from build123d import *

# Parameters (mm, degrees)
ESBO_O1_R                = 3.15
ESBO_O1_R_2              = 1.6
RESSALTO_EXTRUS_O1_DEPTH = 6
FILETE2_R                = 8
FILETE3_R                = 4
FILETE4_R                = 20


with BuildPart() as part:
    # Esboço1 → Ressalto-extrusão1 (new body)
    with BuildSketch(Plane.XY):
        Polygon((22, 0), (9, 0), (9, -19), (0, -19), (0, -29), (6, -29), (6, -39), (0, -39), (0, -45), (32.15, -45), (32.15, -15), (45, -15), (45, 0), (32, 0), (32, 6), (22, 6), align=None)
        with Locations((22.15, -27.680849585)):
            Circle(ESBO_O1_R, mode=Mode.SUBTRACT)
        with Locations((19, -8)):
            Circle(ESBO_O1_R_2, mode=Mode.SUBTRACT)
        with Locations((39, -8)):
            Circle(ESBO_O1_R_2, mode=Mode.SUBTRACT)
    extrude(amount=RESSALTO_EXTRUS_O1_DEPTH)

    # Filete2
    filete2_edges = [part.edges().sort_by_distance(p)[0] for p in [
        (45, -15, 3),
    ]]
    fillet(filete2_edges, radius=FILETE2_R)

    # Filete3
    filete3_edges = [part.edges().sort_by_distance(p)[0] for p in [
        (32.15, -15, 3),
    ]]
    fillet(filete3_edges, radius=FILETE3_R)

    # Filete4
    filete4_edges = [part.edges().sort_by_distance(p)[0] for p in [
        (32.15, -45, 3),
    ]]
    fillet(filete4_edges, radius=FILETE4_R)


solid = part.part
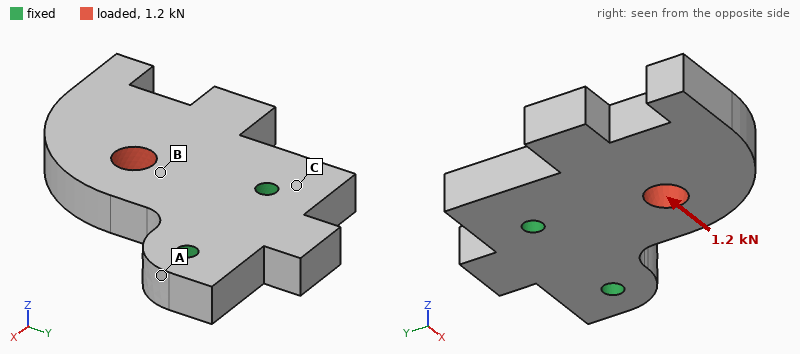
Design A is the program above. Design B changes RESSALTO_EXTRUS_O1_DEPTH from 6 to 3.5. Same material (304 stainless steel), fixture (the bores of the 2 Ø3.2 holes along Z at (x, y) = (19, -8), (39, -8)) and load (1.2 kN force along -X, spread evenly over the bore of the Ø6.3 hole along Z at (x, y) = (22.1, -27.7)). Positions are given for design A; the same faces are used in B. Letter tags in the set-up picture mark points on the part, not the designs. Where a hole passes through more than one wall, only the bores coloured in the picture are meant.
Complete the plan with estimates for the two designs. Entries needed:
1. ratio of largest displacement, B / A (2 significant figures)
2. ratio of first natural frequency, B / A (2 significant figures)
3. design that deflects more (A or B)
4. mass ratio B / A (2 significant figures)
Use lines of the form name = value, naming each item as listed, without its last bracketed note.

ratio of largest displacement, B / A = 1.7
ratio of first natural frequency, B / A = 0.62
design that deflects more = B
mass ratio B / A = 0.58
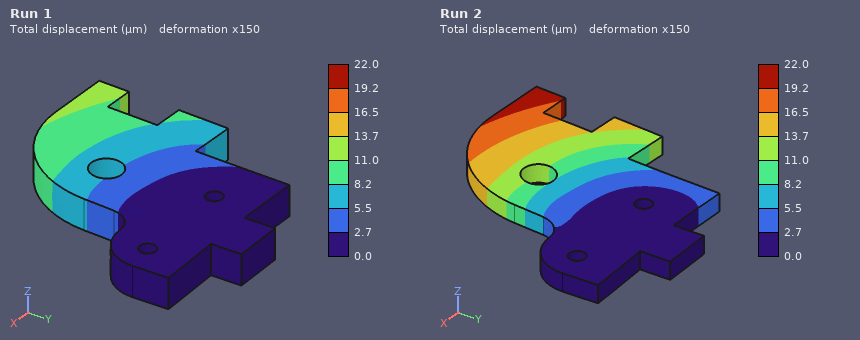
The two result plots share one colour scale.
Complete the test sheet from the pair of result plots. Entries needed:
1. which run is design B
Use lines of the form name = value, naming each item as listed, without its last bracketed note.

which run is design B = Run 2
